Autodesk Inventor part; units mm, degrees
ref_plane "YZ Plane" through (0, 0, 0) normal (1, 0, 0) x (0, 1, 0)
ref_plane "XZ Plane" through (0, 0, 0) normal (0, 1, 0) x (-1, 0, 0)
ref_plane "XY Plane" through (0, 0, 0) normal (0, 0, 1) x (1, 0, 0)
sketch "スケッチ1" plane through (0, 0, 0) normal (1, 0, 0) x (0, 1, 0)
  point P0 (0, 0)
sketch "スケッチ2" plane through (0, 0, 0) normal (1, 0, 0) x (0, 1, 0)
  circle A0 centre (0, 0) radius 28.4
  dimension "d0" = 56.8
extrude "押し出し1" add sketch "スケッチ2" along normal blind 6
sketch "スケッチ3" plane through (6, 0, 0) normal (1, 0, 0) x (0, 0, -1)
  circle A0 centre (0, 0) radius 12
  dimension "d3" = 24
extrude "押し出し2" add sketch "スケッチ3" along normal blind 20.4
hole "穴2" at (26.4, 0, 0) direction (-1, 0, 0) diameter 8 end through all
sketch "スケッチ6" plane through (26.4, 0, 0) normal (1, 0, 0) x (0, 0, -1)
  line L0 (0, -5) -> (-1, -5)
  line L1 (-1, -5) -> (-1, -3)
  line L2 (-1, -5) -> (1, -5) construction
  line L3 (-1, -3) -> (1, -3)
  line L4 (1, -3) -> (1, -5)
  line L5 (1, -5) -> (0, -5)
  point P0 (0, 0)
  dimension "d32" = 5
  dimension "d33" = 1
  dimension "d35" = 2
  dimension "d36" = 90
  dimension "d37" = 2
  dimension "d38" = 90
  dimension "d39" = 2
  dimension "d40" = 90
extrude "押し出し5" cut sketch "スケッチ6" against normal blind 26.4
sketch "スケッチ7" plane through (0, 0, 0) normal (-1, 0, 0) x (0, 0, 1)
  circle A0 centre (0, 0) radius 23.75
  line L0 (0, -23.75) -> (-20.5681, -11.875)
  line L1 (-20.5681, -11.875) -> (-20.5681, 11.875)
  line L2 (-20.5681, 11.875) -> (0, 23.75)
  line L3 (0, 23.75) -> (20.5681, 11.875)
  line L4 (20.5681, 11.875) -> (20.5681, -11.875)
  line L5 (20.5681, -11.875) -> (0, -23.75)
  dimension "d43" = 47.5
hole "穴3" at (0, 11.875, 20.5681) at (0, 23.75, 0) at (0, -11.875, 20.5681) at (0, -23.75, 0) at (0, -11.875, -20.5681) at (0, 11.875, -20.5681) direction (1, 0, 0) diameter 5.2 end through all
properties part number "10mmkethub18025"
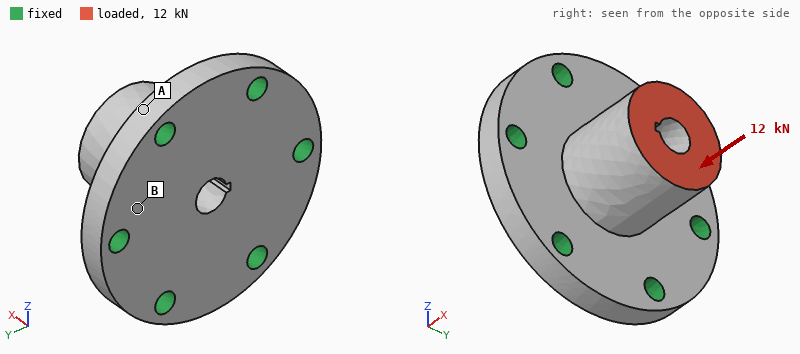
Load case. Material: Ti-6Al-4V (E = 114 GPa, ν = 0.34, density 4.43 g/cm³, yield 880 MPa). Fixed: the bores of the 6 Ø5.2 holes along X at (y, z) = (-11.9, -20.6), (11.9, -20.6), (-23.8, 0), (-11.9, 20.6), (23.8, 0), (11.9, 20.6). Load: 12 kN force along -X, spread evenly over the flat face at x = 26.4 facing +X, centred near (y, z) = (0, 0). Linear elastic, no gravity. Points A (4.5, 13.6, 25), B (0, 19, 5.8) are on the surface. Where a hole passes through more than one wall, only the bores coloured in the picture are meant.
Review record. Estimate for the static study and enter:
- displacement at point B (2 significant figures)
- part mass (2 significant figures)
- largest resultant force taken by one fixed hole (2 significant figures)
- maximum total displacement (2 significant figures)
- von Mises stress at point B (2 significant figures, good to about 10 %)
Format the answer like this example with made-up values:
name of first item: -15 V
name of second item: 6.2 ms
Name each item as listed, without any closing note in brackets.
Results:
displacement at point B: 6.3 µm
part mass: 99 g
largest resultant force taken by one fixed hole: 2.2 kN
maximum total displacement: 26 µm
von Mises stress at point B: 44 MPa
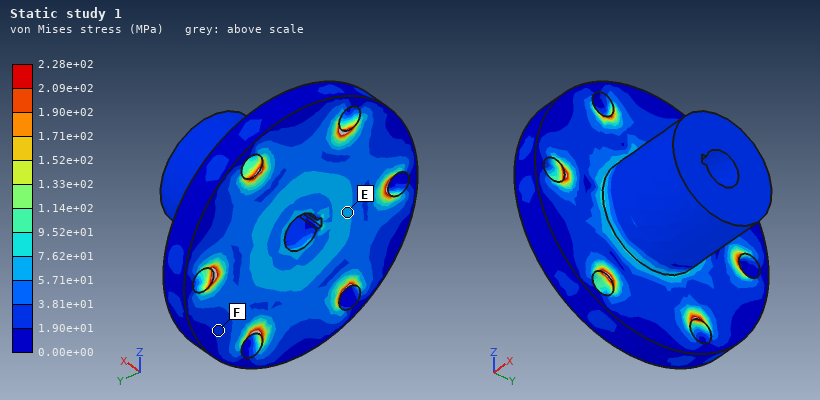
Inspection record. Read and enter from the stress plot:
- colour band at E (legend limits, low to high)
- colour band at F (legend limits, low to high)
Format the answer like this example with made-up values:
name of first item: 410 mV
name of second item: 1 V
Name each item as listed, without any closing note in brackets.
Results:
colour band at E: 5.71e+01 to 7.62e+01 MPa
colour band at F: 1.90e+01 to 3.81e+01 MPa
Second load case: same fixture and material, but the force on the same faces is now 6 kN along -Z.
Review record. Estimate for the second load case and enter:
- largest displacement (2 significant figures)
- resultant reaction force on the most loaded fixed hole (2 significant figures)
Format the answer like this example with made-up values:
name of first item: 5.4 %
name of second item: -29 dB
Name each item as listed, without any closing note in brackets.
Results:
largest displacement: 61 µm
resultant reaction force on the most loaded fixed hole: 2.6 kN
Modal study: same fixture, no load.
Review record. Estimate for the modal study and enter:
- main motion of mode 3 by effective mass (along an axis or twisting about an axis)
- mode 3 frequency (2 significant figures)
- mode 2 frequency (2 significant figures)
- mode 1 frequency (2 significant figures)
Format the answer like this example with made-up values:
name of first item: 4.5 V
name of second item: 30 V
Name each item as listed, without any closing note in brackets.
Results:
main motion of mode 3 by effective mass: along X
mode 3 frequency: 16 kHz
mode 2 frequency: 14 kHz
mode 1 frequency: 13 kHz
